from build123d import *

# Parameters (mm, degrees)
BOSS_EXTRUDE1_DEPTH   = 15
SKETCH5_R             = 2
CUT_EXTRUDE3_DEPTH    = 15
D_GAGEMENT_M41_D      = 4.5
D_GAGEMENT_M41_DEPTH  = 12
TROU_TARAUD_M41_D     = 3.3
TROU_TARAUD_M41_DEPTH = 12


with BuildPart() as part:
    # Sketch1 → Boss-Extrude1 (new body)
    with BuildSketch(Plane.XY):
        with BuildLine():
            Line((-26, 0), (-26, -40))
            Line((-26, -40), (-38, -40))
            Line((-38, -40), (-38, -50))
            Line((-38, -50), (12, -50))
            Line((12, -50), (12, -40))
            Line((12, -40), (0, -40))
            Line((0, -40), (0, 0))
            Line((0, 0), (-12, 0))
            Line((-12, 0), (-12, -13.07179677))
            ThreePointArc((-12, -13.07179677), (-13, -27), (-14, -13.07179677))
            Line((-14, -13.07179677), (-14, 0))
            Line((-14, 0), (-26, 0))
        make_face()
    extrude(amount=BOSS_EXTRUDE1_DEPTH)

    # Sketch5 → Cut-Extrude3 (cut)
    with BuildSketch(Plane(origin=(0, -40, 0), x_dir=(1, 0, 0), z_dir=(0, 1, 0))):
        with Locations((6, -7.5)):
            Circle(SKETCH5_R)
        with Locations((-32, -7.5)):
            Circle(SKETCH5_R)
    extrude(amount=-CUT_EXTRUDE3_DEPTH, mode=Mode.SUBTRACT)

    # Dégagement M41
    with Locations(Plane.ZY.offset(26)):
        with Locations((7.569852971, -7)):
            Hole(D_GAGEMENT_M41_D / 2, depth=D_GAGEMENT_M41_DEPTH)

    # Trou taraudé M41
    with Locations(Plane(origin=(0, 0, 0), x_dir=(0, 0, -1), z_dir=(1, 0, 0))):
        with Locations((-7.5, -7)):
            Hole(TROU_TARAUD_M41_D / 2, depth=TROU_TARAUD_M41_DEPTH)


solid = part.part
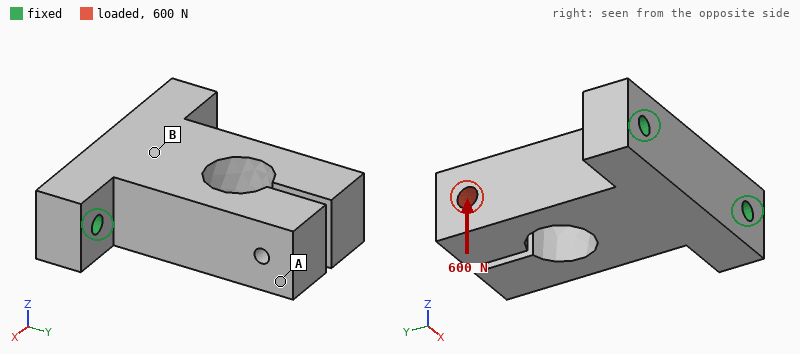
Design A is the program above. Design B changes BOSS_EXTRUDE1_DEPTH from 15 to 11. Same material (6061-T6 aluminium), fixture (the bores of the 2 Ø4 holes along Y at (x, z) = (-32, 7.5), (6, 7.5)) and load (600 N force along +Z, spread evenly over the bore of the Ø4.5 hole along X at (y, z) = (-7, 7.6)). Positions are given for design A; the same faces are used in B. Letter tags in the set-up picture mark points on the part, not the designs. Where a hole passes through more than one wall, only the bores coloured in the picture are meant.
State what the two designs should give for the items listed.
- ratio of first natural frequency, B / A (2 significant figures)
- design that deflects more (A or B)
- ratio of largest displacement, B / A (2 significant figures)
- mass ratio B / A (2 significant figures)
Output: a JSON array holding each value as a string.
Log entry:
["0.86", "B", "2.0", "0.73"]
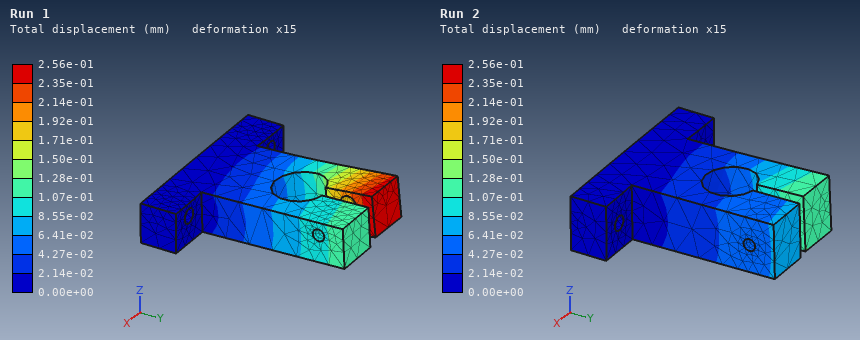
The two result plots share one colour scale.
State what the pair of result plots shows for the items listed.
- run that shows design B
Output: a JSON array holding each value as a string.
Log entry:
["Run 1"]
